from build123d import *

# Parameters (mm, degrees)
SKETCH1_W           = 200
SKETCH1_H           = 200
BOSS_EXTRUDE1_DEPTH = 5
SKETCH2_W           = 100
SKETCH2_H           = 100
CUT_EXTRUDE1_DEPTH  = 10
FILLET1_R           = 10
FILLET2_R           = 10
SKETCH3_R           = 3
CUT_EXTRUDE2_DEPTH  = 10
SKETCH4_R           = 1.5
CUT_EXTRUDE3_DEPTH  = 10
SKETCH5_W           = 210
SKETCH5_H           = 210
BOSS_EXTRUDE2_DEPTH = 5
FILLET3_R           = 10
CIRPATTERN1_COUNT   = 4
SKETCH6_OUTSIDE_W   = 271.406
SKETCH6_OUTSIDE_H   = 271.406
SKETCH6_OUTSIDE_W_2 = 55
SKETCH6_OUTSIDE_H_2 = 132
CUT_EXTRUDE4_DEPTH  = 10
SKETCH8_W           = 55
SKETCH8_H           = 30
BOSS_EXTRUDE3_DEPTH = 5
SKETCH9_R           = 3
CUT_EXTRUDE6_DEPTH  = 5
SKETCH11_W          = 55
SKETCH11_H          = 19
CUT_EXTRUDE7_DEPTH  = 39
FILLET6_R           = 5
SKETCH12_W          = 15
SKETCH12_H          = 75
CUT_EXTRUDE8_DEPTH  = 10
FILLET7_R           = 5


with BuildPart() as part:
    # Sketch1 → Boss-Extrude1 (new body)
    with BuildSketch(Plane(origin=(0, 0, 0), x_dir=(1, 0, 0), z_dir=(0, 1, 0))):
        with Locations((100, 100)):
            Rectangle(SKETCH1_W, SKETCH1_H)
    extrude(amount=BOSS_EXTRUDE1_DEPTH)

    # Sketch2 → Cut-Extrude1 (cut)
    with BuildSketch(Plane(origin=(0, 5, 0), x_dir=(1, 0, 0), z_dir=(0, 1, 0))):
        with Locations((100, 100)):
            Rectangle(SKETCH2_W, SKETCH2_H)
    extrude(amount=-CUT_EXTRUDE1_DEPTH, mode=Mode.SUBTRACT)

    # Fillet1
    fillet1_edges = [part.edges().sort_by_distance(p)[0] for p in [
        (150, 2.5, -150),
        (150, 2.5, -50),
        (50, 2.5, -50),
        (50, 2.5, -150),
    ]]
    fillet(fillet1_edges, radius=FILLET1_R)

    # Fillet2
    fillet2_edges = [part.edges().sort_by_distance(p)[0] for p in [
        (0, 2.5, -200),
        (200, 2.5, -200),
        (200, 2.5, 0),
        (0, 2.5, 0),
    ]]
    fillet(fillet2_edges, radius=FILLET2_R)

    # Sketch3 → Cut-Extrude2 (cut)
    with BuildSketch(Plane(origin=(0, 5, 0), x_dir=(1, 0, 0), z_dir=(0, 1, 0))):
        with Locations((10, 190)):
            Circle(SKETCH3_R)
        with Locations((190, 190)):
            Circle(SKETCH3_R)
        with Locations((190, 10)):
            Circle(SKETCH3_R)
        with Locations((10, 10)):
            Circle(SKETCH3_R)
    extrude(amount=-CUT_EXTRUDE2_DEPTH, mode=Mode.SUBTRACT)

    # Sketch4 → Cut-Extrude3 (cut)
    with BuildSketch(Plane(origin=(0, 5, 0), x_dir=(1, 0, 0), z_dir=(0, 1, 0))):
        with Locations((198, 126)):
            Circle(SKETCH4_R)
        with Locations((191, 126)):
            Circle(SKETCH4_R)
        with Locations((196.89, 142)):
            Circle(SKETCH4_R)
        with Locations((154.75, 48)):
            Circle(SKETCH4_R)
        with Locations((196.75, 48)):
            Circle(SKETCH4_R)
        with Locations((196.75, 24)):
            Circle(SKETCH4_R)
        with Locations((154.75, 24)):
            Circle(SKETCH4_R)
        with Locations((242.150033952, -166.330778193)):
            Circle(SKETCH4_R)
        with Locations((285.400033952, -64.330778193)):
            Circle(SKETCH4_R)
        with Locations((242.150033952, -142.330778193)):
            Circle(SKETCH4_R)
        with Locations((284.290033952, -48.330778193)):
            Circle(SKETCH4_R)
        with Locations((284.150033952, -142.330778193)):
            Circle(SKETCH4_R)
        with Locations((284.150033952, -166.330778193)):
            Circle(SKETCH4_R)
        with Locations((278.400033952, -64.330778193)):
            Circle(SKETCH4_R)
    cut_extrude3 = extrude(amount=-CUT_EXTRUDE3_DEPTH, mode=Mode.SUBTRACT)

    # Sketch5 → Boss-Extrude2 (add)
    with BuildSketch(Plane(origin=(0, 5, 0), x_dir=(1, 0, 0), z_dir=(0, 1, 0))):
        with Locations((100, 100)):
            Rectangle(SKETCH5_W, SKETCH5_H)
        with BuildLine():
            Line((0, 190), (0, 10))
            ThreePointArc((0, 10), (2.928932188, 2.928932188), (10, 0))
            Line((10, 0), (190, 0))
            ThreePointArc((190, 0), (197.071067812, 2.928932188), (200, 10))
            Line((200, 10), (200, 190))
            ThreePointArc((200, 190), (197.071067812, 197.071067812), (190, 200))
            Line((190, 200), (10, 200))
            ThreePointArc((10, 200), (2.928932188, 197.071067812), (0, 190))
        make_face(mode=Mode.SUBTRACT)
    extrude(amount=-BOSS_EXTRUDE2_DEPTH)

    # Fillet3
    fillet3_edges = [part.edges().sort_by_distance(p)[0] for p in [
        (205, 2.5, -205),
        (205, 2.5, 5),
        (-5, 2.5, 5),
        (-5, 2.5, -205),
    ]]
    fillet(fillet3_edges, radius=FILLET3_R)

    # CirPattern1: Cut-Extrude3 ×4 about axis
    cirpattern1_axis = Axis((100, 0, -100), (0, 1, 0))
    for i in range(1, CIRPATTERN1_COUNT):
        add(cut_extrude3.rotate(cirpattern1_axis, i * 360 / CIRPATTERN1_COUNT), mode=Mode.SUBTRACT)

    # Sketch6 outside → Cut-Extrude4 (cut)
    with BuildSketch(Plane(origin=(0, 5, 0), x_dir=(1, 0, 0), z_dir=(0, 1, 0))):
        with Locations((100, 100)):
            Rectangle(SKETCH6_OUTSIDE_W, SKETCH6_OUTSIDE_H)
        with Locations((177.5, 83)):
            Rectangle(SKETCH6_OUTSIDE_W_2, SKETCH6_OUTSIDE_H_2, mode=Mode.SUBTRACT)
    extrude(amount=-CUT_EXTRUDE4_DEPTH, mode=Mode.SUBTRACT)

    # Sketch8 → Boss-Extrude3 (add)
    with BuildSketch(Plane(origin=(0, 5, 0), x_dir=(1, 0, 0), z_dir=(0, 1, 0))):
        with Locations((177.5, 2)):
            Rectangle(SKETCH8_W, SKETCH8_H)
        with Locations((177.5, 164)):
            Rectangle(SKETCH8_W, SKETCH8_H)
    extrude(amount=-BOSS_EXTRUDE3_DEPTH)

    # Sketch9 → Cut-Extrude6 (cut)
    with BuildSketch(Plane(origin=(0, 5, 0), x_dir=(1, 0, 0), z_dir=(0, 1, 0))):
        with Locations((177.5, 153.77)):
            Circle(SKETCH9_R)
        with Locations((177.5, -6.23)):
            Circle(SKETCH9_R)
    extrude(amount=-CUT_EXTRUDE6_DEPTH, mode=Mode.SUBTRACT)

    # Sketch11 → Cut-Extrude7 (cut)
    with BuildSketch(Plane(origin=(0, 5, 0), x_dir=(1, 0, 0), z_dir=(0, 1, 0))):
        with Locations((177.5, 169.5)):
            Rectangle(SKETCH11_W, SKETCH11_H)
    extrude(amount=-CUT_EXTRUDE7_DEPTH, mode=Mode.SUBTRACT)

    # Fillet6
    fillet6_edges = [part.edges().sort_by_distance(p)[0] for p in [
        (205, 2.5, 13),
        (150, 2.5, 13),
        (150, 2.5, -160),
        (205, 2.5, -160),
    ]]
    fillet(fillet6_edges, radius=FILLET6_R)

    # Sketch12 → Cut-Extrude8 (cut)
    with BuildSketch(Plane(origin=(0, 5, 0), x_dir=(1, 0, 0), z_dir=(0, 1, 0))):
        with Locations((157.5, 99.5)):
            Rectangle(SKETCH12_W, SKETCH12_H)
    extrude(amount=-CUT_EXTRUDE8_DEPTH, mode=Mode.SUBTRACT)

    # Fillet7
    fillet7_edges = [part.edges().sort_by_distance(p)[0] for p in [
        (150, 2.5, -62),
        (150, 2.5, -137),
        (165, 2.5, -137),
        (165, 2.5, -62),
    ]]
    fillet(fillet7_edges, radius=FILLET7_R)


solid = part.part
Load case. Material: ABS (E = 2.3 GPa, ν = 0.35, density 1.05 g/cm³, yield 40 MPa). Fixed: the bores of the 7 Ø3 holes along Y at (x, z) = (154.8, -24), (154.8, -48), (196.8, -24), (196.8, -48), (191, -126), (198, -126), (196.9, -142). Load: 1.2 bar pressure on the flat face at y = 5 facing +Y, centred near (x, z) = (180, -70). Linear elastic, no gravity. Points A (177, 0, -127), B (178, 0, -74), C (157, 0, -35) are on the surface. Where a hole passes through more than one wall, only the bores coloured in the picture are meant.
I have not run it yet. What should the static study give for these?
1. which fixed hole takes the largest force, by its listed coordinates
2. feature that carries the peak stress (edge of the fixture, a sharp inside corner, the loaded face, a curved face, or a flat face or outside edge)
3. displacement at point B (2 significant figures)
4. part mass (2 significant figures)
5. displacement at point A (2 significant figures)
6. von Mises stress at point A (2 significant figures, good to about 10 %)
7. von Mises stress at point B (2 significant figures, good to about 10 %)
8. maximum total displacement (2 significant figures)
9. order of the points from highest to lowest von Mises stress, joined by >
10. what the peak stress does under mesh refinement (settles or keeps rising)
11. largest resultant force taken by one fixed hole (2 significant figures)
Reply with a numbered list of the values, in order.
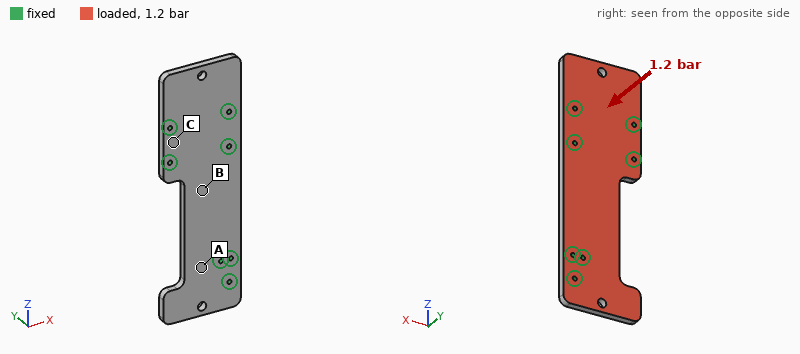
1. (191, -126)
2. edge of the fixture
3. 0.54 mm
4. 43 g
5. 0.39 mm
6. 9.3 MPa
7. 5.0 MPa
8. 2.0 mm
9. A > B > C
10. keeps rising
11. 350 N
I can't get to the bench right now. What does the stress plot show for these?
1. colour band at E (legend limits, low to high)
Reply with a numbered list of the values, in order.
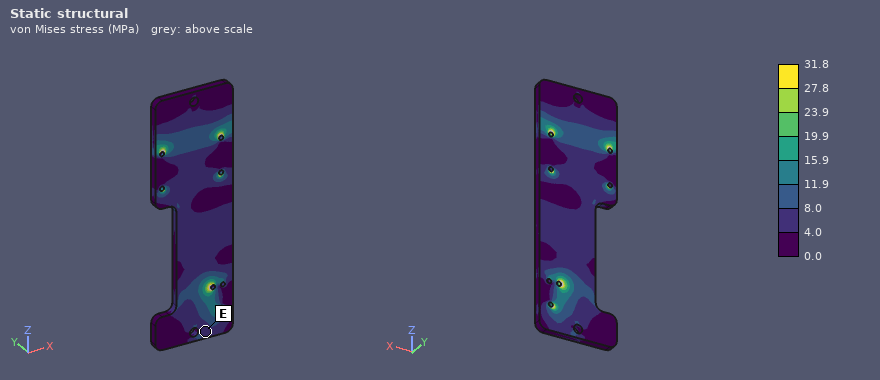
1. 4.0 to 8.0 MPa
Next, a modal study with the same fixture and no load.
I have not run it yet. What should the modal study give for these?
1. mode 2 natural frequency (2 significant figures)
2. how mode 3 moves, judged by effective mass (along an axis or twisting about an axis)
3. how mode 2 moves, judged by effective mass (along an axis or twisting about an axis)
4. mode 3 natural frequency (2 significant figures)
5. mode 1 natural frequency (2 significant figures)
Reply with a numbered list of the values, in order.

1. 780 Hz
2. along Y
3. along Y
4. 1100 Hz
5. 700 Hz
